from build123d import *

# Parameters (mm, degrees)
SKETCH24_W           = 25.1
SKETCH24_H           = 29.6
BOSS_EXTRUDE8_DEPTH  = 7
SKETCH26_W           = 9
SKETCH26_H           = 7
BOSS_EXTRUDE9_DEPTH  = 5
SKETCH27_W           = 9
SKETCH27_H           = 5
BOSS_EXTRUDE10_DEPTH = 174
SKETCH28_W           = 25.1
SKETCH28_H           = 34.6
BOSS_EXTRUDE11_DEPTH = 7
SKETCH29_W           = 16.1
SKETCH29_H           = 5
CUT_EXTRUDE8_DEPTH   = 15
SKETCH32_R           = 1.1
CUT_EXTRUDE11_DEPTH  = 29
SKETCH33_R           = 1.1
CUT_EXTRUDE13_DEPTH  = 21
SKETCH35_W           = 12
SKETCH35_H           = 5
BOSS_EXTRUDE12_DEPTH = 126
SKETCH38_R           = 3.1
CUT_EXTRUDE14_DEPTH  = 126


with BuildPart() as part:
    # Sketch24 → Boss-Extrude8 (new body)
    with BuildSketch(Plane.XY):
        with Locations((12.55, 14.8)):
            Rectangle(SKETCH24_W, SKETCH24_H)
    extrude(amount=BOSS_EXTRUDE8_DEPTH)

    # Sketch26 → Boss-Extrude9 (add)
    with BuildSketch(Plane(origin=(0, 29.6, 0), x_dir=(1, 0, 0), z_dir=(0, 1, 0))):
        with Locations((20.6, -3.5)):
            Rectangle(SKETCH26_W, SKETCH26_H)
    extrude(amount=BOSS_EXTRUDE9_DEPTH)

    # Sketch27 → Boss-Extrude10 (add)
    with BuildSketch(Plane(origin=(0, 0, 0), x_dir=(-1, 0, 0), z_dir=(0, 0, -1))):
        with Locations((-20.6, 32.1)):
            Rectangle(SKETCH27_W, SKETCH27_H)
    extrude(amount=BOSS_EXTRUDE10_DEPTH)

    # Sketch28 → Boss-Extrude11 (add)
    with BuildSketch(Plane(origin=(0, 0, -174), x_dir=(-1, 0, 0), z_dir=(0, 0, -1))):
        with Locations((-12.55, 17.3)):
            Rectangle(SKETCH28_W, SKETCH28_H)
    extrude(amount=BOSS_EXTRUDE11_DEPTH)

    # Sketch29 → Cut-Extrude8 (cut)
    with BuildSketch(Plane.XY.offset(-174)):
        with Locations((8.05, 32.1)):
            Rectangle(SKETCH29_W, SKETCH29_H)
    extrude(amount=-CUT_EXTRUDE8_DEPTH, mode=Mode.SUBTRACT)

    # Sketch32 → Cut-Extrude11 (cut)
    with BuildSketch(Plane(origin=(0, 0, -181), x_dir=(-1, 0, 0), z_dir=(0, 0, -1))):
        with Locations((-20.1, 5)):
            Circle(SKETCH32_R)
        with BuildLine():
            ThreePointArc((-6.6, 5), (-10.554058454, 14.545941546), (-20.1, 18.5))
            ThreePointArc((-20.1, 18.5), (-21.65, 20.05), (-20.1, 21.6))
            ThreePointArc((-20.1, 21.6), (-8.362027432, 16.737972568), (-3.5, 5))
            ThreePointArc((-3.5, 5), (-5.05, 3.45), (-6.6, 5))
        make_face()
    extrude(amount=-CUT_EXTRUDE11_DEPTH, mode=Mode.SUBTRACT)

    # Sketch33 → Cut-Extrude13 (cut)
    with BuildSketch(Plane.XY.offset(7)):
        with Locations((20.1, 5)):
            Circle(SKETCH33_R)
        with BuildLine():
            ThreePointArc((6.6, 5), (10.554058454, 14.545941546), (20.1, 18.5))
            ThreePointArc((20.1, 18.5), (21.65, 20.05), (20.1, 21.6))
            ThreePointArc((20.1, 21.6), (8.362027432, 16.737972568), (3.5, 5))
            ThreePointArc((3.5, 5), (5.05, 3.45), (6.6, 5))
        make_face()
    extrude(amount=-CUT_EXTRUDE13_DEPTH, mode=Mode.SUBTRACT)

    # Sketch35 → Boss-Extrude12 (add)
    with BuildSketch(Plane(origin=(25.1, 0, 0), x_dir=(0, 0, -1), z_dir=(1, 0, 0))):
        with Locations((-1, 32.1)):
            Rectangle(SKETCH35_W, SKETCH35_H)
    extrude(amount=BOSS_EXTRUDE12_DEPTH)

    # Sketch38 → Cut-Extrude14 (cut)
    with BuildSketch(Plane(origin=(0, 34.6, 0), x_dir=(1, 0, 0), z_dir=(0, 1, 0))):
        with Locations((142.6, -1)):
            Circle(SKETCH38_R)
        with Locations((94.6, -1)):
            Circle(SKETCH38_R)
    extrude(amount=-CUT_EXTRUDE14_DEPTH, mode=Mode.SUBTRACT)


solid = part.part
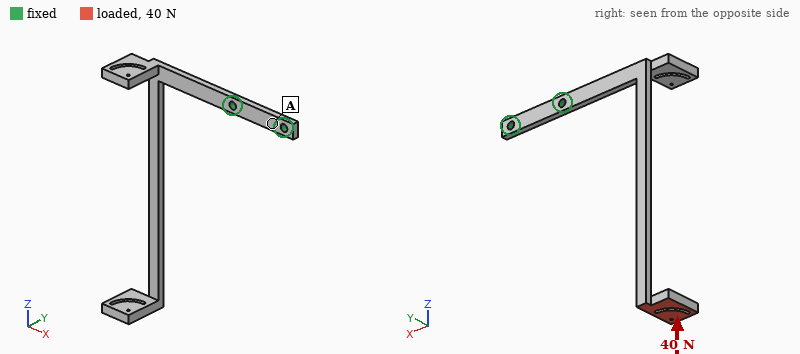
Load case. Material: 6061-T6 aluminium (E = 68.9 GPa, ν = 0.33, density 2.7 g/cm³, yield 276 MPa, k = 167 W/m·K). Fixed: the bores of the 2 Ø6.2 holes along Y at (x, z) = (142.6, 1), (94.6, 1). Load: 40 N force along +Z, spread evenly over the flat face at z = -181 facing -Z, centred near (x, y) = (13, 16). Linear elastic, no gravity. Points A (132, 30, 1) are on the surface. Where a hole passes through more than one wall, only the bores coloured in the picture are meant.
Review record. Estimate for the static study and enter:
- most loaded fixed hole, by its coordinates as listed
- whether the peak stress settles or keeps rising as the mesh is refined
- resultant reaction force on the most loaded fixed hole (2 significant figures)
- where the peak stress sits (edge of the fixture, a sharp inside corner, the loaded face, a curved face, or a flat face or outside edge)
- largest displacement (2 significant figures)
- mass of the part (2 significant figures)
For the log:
(94.6, 1)
keeps rising
48 N
edge of the fixture
2.7 mm
67 g
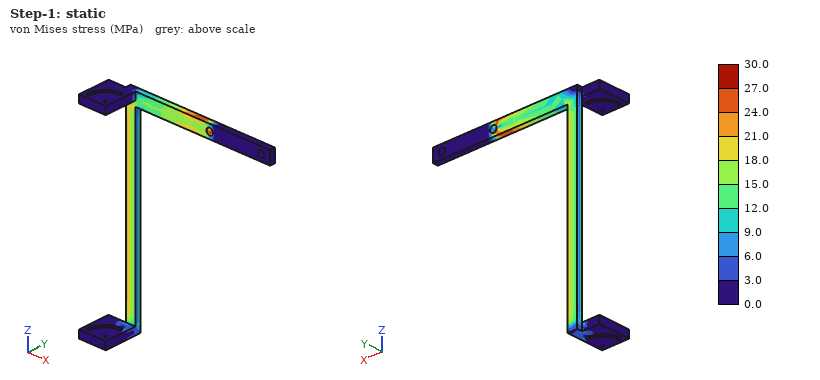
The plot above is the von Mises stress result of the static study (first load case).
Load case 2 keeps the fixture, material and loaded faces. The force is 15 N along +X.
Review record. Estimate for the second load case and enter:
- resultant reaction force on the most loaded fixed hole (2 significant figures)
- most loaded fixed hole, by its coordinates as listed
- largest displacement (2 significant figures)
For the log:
16 N
(94.6, 1)
2.4 mm
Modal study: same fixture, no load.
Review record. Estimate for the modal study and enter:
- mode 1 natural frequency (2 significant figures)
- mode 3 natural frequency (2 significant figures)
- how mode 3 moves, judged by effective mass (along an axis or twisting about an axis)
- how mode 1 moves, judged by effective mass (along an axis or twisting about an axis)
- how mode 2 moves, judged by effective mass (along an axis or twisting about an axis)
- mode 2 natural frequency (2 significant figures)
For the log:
50 Hz
240 Hz
along Y
along Y
along X
98 Hz
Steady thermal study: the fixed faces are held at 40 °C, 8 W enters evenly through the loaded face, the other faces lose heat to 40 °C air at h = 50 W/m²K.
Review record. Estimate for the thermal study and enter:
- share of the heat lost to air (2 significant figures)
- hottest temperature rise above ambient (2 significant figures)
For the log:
97 %
44 K
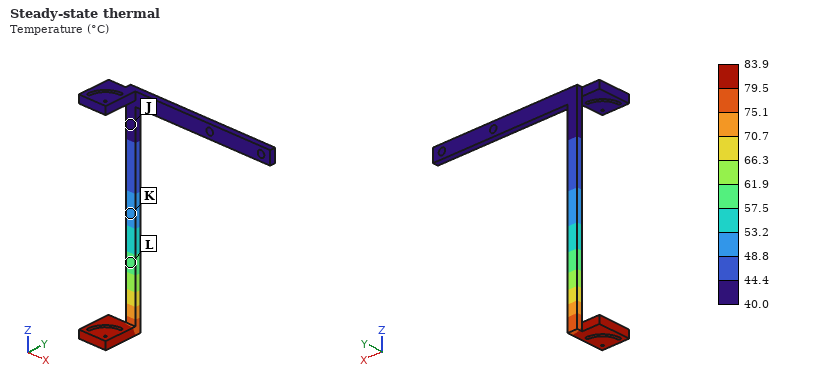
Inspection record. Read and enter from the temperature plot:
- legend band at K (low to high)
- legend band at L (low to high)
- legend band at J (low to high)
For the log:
48.8 to 53.2 °C
57.5 to 61.9 °C
40.0 to 44.4 °C
